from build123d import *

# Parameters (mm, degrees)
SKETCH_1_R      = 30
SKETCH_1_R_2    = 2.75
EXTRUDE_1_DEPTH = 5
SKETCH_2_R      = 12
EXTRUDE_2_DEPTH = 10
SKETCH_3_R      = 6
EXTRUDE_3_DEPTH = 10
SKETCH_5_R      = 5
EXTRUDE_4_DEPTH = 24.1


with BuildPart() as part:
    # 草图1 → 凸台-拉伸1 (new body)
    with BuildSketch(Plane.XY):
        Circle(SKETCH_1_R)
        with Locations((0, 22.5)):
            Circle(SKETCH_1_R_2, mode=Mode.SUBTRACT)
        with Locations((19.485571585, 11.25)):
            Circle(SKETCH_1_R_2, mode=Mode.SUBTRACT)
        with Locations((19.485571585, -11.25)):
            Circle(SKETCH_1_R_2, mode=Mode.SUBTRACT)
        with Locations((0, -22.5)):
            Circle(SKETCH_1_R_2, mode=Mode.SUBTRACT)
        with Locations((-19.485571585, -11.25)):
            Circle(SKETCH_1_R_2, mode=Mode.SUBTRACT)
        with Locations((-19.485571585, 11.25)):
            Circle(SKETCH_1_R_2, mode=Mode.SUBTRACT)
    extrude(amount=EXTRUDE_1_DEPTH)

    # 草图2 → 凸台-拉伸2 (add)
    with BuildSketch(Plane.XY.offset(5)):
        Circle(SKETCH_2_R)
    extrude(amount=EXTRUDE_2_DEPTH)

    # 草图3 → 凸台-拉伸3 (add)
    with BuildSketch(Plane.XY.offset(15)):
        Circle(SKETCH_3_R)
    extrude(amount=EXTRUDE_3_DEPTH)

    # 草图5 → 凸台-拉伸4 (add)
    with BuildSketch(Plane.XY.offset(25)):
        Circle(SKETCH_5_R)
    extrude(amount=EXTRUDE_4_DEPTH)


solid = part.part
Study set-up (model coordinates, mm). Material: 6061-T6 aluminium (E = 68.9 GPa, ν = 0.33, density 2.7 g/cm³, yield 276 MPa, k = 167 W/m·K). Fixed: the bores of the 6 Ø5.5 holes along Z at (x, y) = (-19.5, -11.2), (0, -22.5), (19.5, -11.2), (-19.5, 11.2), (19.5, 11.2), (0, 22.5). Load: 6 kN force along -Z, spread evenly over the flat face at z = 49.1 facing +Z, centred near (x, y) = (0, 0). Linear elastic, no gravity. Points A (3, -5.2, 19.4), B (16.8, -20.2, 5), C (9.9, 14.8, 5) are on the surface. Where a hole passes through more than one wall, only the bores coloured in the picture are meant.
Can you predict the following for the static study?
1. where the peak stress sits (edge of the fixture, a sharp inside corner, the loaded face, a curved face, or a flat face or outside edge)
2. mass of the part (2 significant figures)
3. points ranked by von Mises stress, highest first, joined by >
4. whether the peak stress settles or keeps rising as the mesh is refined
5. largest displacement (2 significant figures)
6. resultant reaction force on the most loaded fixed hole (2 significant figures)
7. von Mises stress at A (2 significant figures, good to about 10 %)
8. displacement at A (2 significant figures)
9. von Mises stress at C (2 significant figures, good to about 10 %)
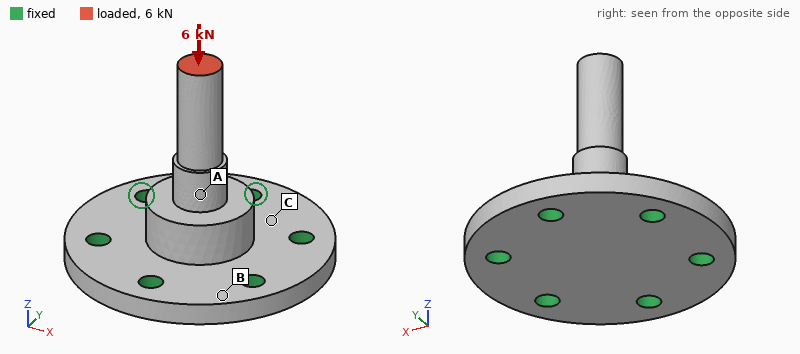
edge of the fixture
57 g
A > C > B
keeps rising
58 µm
1.1 kN
50 MPa
26 µm
23 MPa
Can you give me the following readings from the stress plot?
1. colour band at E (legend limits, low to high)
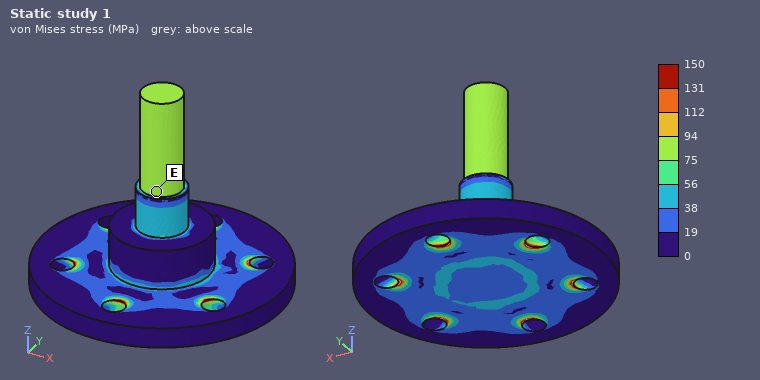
75 to 94 MPa
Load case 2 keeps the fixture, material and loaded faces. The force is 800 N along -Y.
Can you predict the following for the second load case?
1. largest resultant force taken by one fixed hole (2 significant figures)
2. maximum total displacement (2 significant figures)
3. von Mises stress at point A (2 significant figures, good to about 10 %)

740 N
0.31 mm
120 MPa
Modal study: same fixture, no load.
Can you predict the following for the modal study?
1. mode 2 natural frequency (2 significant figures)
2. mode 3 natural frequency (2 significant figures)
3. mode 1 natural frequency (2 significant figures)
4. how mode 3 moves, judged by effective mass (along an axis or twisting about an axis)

5800 Hz
16 kHz
5800 Hz
along Z
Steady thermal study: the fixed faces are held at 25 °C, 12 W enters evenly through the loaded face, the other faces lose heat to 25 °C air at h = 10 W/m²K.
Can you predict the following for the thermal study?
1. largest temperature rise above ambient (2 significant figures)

33 K
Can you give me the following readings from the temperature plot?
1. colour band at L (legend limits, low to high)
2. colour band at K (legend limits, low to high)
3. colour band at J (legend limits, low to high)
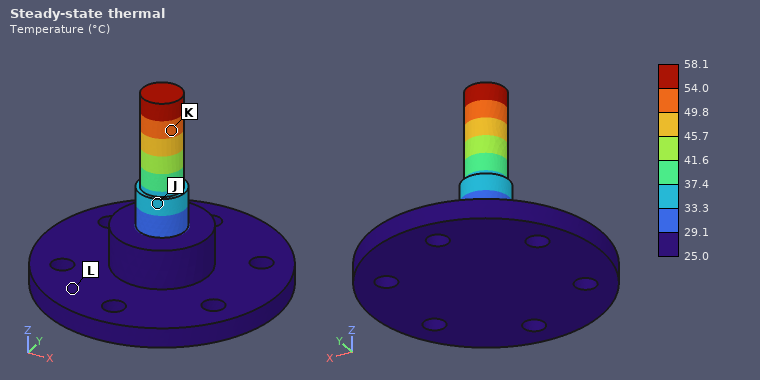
25.0 to 29.1 °C
49.8 to 54.0 °C
33.3 to 37.4 °C
